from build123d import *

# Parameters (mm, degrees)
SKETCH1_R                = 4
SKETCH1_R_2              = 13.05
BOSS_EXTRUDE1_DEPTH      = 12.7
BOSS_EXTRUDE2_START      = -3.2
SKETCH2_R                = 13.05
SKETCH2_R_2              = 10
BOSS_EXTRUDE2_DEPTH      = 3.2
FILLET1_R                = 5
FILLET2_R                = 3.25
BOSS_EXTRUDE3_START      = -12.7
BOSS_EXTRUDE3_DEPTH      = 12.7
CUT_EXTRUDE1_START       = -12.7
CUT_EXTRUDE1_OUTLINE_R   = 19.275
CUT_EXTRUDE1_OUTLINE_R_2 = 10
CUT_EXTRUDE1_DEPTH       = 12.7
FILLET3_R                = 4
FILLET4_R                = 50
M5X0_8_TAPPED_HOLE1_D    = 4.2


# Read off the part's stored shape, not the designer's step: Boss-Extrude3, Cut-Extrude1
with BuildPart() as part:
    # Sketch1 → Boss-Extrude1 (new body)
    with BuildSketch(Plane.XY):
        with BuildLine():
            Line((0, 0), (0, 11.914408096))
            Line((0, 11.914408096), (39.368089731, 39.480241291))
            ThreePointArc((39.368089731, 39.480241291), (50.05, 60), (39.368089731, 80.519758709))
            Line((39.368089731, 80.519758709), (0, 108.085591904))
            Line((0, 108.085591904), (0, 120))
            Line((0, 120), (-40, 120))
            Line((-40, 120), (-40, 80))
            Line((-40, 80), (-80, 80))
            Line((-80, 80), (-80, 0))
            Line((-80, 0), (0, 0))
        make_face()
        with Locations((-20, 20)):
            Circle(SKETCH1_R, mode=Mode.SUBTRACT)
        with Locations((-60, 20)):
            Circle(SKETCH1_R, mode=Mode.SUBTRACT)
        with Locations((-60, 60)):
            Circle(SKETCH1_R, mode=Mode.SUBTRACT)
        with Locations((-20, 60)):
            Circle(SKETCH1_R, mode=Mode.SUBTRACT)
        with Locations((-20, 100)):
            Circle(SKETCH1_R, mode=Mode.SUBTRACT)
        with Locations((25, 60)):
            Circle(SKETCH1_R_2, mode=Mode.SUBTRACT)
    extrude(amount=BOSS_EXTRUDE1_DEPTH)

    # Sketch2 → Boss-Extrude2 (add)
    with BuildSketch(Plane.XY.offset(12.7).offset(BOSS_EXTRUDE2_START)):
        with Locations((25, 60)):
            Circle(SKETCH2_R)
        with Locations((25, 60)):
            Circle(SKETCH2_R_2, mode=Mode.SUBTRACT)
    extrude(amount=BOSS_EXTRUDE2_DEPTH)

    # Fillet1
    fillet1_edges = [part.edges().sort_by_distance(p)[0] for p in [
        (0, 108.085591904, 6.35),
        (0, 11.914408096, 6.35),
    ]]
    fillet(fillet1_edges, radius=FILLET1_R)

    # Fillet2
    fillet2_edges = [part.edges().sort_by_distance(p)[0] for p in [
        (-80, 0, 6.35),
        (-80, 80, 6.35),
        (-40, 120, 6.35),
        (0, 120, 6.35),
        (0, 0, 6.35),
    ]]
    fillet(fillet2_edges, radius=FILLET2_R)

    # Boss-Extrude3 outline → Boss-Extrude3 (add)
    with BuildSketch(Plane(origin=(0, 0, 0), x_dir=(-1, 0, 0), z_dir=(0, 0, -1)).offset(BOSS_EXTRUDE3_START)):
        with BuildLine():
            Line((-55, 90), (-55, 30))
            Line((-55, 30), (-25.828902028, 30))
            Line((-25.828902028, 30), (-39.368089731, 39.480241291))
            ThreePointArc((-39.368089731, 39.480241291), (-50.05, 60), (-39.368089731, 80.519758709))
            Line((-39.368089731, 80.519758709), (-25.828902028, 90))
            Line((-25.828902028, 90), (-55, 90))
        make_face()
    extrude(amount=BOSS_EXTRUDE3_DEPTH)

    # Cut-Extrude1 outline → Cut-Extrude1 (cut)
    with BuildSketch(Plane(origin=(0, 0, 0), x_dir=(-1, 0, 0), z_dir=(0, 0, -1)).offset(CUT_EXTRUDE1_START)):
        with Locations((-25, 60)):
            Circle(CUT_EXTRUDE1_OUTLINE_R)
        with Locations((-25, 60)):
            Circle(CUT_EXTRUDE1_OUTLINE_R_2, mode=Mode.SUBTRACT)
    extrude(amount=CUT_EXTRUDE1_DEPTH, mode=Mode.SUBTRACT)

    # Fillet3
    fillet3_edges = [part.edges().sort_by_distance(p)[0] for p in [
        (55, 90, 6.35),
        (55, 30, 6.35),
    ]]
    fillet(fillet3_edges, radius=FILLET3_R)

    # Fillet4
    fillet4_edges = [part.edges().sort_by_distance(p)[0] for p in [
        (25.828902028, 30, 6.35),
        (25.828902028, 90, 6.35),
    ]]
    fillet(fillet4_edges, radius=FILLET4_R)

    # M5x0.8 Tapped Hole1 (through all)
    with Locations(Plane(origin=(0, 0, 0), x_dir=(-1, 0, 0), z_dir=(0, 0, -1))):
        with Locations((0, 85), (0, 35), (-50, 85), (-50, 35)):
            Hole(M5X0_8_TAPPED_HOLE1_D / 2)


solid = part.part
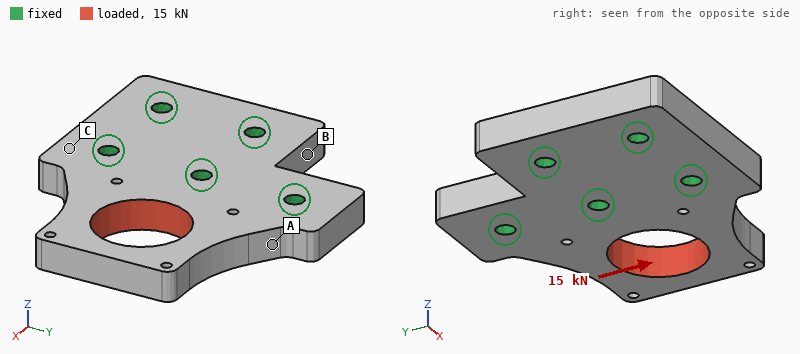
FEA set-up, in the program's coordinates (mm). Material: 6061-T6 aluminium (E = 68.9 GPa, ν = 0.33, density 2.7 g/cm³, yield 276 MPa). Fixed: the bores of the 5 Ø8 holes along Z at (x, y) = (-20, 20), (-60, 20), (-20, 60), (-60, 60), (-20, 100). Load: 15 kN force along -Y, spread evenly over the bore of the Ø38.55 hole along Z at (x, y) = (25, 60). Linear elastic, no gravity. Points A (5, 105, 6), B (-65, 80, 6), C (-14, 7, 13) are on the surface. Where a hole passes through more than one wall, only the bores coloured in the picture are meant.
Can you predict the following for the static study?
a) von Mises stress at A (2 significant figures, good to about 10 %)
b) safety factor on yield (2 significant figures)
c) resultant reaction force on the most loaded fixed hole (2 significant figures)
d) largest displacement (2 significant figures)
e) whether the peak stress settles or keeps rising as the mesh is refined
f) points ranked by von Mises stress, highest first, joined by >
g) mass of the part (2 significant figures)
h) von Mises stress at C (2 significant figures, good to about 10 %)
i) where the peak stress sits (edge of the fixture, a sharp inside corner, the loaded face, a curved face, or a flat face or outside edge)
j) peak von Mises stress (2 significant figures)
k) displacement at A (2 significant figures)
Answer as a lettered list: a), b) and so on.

a) 43 MPa
b) 3.3
c) 8.9 kN
d) 99 µm
e) settles
f) A > C > B
g) 350 g
h) 16 MPa
i) the loaded face
j) 84 MPa
k) 17 µm
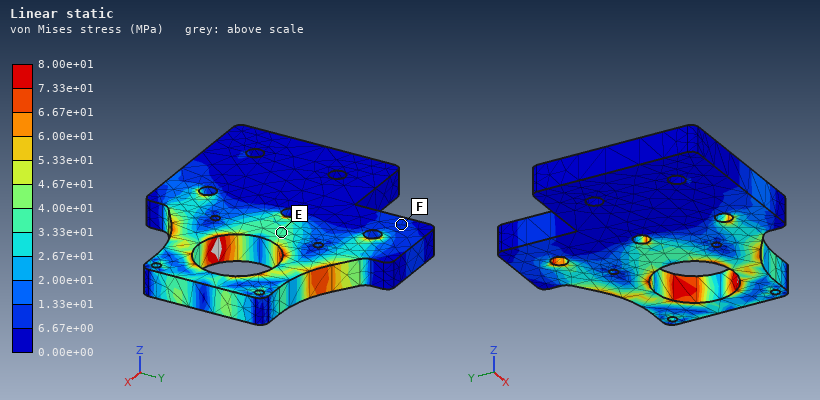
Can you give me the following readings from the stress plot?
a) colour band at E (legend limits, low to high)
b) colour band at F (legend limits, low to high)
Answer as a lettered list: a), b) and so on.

a) 3.33e+01 to 4.00e+01 MPa
b) 6.67e+00 to 1.33e+01 MPa
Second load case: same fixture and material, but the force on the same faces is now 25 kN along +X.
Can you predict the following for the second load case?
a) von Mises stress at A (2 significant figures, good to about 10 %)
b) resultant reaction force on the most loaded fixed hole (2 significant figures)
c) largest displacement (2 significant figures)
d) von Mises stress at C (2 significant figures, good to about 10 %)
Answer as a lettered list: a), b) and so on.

a) 21 MPa
b) 8.4 kN
c) 56 µm
d) 8.7 MPa
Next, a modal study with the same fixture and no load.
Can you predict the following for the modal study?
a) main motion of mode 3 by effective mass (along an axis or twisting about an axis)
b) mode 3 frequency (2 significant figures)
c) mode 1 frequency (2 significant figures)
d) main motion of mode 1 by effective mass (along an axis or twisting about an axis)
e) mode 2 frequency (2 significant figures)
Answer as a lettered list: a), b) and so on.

a) along Y
b) 7400 Hz
c) 2200 Hz
d) along Z
e) 4900 Hz
